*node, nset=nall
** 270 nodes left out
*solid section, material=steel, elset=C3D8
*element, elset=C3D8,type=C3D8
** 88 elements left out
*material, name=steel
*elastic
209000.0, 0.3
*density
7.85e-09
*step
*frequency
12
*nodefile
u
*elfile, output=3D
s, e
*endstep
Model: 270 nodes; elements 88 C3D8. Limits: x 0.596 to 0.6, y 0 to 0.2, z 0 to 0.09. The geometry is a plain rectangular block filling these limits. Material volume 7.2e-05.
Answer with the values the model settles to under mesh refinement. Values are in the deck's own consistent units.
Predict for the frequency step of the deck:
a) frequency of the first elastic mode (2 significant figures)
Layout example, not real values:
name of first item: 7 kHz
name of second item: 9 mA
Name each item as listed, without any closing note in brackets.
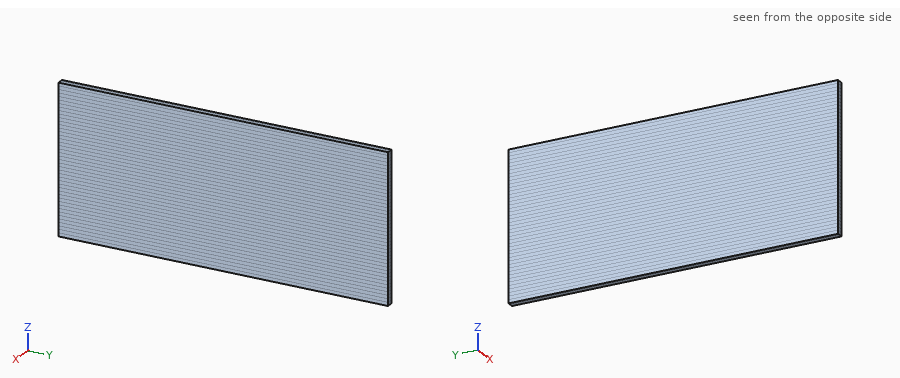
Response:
frequency of the first elastic mode: 6.3e+05 cycles per unit time
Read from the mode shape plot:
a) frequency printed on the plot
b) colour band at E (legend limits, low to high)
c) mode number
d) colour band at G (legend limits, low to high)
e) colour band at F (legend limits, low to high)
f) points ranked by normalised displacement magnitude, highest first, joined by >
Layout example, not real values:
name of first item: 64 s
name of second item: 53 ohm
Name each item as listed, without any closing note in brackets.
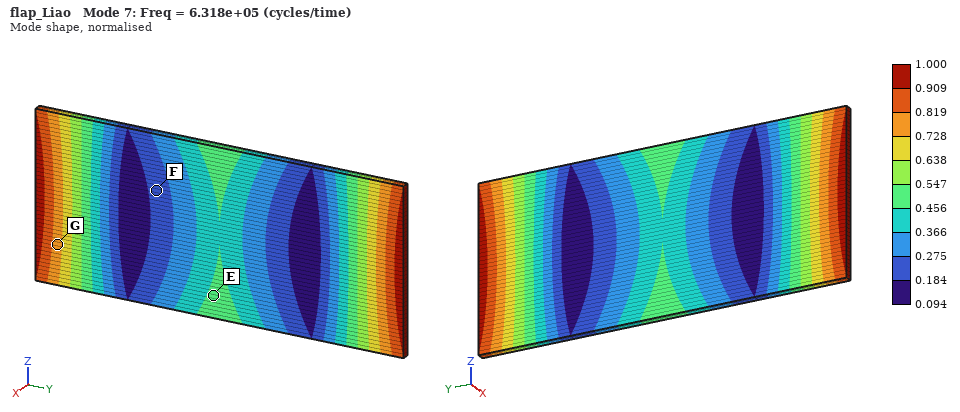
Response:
frequency printed on the plot: 6.318e+05
colour band at E: 0.456 to 0.547
mode number: 7
colour band at G: 0.728 to 0.819
colour band at F: 0.184 to 0.275
points ranked by normalised displacement magnitude, highest first, joined by >: G > E > F
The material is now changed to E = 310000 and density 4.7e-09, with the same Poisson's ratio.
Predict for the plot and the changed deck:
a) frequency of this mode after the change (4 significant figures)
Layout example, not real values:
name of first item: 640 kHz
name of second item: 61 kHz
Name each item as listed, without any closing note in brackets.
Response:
frequency of this mode after the change: 9.945e+05
